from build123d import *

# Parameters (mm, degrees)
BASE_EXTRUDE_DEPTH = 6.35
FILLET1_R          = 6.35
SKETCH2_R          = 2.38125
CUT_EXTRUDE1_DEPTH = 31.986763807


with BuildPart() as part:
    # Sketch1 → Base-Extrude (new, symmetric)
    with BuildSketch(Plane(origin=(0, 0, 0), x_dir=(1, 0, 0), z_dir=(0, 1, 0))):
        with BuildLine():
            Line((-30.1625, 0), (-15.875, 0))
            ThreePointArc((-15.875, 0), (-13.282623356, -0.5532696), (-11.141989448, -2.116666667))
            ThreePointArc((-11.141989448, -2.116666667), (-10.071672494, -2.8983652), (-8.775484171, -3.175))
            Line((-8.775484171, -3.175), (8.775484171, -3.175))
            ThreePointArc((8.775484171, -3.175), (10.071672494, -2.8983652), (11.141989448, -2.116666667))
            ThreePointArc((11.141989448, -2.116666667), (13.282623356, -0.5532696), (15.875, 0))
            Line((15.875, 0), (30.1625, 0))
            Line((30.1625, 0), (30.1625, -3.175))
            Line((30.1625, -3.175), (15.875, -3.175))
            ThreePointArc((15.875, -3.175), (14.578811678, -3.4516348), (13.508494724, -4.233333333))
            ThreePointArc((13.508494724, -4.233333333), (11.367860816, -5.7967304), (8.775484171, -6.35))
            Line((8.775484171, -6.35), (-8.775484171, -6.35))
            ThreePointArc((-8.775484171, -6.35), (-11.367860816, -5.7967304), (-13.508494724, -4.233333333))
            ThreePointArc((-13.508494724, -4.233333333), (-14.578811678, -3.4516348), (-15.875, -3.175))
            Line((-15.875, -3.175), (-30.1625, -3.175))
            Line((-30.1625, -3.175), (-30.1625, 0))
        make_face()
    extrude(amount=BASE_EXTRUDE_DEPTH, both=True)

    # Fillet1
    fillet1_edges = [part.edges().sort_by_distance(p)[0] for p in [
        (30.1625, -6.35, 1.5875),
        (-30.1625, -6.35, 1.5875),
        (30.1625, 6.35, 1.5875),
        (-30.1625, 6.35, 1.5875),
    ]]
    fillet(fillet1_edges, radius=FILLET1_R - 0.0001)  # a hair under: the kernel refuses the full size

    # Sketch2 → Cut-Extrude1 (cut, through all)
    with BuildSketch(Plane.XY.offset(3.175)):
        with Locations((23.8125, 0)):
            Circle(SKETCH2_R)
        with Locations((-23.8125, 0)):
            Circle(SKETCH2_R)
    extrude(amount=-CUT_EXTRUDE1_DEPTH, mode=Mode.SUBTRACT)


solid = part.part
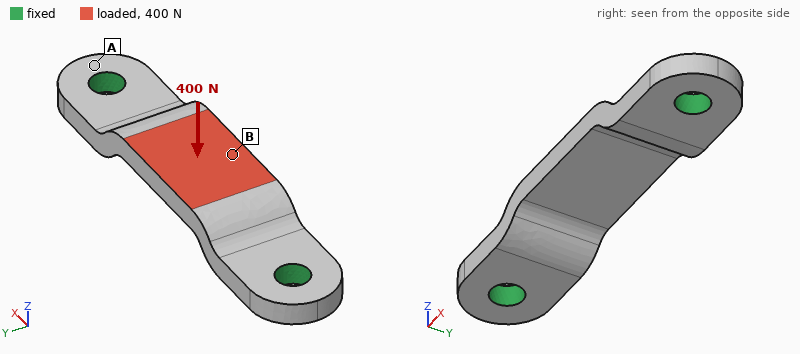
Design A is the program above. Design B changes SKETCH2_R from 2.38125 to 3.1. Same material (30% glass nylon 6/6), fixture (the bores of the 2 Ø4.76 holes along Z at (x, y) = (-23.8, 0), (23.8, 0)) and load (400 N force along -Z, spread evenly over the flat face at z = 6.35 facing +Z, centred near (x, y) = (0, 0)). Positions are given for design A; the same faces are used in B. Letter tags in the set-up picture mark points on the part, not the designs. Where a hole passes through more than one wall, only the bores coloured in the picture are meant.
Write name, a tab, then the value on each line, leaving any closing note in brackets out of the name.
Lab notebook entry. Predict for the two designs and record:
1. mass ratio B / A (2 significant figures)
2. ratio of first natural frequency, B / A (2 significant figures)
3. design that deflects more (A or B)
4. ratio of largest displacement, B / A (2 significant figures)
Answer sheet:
mass ratio B / A	0.97
ratio of first natural frequency, B / A	1.1
design that deflects more	A
ratio of largest displacement, B / A	0.89
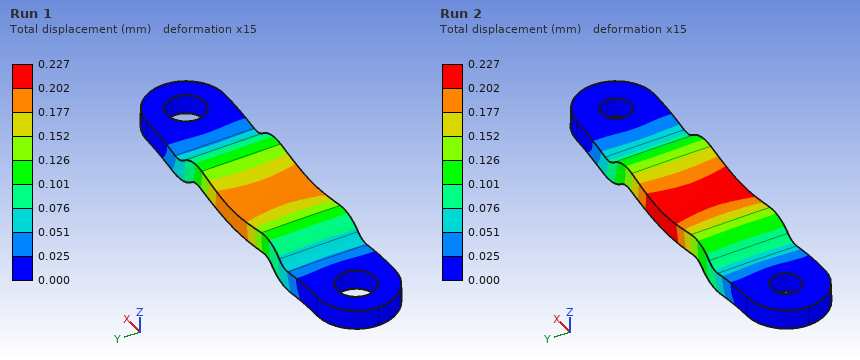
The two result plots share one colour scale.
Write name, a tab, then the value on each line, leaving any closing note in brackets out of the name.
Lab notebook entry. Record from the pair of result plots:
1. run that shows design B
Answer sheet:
run that shows design B	Run 1
